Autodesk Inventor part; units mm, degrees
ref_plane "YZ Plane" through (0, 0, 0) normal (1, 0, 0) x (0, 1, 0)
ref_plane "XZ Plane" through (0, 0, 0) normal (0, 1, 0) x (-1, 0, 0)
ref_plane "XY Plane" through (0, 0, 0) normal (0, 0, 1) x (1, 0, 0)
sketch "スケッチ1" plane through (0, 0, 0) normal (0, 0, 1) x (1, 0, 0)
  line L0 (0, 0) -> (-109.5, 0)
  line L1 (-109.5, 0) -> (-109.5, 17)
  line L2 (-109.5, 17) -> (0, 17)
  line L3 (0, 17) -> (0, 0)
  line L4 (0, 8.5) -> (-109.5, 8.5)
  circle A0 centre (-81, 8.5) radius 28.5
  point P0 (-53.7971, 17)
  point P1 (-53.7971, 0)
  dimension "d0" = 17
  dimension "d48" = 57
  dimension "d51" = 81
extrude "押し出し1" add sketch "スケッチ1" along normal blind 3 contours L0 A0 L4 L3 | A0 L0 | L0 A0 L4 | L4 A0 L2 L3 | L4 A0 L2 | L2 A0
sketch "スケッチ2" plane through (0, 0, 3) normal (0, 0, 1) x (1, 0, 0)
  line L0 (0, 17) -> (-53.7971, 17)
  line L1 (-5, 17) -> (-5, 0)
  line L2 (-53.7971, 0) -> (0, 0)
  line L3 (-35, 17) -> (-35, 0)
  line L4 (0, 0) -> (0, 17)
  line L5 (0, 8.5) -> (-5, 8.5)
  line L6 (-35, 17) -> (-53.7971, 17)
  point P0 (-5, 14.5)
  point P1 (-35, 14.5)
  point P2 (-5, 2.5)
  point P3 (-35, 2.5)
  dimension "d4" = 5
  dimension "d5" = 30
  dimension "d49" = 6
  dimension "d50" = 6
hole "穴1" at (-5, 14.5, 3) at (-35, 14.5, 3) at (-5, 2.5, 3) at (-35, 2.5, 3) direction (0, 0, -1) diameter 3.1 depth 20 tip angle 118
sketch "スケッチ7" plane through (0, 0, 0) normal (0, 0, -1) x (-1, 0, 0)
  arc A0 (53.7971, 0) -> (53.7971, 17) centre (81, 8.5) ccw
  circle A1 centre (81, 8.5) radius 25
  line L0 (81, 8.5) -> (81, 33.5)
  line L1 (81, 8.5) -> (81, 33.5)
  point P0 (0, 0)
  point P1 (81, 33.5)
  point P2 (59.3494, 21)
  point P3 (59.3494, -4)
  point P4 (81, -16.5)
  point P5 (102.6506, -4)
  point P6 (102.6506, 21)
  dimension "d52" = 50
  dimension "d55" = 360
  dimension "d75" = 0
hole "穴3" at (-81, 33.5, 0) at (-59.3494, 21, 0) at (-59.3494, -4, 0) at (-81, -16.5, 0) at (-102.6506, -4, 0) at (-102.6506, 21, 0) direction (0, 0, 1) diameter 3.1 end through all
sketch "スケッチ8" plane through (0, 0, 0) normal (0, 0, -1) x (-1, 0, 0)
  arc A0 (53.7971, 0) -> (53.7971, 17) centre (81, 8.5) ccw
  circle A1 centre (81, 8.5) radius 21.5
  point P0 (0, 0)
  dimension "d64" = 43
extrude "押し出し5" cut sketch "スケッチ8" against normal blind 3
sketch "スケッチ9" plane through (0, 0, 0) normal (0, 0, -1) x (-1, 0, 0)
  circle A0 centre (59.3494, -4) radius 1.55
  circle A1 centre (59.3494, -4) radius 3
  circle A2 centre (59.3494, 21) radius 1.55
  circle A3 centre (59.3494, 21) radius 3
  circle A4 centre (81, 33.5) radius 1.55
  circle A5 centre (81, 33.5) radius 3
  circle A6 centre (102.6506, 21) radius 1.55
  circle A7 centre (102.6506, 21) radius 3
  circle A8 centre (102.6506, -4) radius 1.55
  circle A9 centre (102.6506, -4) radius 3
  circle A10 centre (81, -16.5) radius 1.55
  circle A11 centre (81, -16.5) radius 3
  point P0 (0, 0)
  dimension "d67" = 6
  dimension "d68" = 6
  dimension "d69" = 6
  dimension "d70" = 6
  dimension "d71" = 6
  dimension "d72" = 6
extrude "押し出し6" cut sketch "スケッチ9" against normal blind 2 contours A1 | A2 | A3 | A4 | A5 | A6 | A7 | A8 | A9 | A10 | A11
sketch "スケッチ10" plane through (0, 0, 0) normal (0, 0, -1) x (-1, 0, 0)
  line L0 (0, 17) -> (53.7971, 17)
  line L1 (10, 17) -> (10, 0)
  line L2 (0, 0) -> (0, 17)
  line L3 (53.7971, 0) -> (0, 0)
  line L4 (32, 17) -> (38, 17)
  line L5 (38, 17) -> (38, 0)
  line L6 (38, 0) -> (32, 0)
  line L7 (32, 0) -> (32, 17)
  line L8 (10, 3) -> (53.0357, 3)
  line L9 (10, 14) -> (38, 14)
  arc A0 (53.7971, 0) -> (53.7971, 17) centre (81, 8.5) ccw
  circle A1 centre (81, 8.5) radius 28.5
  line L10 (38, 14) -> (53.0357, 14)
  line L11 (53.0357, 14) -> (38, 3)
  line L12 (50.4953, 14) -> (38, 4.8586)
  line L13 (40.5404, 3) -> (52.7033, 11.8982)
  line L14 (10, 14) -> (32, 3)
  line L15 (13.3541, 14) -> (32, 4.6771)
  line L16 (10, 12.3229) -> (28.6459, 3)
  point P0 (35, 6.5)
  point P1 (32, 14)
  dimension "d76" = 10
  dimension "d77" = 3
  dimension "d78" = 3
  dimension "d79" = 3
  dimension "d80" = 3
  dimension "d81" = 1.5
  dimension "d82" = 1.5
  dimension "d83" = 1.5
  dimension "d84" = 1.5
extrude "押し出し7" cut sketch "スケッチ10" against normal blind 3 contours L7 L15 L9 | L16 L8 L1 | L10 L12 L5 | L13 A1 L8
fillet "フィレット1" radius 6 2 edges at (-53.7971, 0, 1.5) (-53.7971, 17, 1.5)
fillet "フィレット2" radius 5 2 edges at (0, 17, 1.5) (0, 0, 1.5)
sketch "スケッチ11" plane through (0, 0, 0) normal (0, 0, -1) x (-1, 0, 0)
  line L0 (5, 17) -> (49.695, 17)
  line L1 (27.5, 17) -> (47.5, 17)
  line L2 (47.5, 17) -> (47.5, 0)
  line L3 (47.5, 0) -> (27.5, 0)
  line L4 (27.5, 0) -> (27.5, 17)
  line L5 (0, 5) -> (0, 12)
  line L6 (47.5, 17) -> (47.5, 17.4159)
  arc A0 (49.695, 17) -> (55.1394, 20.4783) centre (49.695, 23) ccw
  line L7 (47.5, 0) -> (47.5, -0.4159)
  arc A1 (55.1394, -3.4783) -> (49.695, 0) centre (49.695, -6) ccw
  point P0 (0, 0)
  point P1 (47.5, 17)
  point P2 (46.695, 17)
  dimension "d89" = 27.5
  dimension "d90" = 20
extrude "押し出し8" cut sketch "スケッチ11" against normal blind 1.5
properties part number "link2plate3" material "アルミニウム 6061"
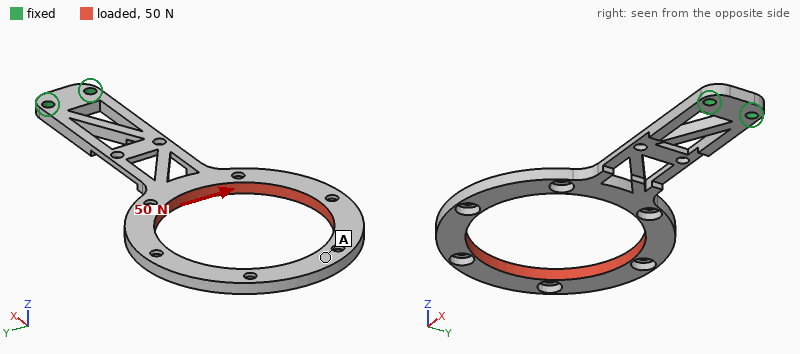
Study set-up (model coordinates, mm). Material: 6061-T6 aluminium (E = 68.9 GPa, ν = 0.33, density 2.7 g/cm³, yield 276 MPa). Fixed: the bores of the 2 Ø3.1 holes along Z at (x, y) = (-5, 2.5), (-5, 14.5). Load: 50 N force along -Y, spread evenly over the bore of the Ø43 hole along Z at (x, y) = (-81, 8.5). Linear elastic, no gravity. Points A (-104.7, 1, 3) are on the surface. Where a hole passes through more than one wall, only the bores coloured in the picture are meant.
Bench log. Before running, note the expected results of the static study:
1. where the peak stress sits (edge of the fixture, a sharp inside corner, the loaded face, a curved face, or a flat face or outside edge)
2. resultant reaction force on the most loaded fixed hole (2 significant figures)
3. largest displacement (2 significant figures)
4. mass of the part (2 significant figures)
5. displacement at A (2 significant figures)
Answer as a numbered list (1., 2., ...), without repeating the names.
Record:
1. a curved face
2. 280 N
3. 0.37 mm
4. 12 g
5. 0.34 mm
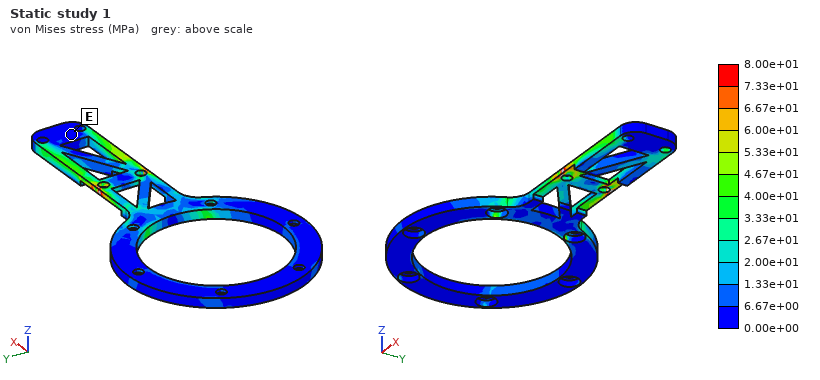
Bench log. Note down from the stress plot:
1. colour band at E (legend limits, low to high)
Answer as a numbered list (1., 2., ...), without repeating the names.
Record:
1. 0.00e+00 to 6.67e+00 MPa
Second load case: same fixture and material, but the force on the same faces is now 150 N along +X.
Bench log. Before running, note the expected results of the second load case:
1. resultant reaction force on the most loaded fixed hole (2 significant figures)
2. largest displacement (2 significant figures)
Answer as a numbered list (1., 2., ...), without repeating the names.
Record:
1. 77 N
2. 1.2 mm
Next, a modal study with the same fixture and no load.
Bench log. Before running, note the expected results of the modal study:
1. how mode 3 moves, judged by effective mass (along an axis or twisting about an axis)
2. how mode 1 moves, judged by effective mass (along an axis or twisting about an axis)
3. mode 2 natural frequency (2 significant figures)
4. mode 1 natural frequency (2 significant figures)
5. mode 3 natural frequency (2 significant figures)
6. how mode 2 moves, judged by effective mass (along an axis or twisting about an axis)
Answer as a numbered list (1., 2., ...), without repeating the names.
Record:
1. along Y
2. along Z
3. 320 Hz
4. 89 Hz
5. 750 Hz
6. twisting about X
